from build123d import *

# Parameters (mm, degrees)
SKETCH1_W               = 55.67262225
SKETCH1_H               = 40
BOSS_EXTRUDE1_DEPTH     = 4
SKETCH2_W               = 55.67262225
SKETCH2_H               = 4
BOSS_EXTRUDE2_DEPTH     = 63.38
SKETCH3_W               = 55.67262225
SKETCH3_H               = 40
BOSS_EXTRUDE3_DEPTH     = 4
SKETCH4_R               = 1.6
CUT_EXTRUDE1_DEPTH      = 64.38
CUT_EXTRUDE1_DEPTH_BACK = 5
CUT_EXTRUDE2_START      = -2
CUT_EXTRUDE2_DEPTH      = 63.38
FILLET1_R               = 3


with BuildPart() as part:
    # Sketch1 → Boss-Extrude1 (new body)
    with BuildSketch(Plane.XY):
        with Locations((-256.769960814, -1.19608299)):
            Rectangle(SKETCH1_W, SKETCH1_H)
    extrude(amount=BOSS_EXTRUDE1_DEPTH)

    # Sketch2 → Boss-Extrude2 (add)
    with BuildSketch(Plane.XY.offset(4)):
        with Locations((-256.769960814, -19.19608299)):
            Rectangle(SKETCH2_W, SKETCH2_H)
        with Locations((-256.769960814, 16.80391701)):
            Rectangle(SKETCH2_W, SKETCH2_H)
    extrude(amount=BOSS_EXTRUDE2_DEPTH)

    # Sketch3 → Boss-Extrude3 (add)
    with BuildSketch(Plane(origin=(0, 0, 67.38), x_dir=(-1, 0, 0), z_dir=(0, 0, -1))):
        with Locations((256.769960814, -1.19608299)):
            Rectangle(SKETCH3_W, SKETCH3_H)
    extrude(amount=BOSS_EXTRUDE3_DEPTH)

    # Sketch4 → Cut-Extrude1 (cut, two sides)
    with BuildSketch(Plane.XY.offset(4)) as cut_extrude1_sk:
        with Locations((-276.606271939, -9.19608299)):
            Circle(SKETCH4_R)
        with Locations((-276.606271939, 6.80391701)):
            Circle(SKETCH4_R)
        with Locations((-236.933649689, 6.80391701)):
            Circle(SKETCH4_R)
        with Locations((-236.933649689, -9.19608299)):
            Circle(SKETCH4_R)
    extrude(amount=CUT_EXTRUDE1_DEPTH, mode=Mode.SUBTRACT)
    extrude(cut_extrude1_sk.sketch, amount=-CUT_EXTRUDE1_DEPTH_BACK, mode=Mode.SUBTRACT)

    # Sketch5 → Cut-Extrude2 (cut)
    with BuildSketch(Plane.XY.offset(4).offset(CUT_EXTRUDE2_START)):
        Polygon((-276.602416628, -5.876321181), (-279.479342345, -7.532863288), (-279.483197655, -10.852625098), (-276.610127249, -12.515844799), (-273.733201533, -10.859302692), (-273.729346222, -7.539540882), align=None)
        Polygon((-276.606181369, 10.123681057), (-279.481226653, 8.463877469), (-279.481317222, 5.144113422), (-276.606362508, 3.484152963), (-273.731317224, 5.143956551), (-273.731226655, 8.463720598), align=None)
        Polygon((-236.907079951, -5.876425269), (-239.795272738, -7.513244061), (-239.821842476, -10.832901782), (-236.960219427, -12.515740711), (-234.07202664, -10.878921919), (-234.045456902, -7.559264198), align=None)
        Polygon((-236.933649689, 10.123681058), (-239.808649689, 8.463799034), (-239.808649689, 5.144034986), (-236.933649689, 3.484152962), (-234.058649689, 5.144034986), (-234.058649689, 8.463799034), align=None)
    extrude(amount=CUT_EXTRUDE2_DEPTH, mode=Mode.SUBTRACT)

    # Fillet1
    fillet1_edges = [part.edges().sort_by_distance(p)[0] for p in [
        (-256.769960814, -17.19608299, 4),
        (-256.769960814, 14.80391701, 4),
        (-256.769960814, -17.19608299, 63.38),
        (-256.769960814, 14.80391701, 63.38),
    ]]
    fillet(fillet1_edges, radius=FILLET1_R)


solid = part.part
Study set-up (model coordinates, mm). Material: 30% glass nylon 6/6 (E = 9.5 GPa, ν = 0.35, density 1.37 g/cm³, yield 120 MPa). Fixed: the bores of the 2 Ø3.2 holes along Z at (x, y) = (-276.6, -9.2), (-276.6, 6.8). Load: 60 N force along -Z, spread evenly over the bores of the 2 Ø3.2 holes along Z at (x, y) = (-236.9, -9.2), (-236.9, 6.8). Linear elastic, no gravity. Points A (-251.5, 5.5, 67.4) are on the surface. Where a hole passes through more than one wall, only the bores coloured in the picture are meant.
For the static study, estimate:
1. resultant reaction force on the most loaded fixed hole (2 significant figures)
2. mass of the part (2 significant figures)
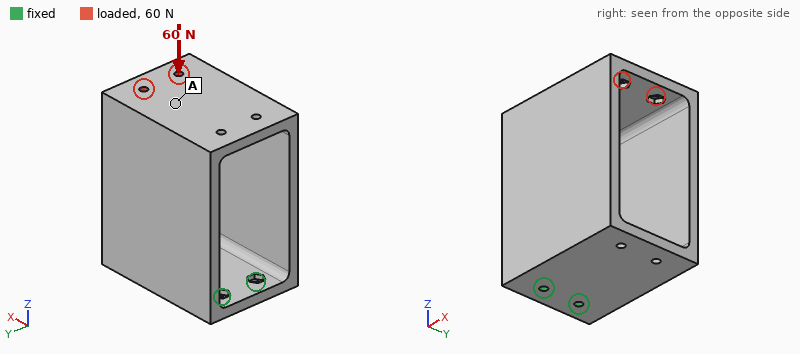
32 N
60 g
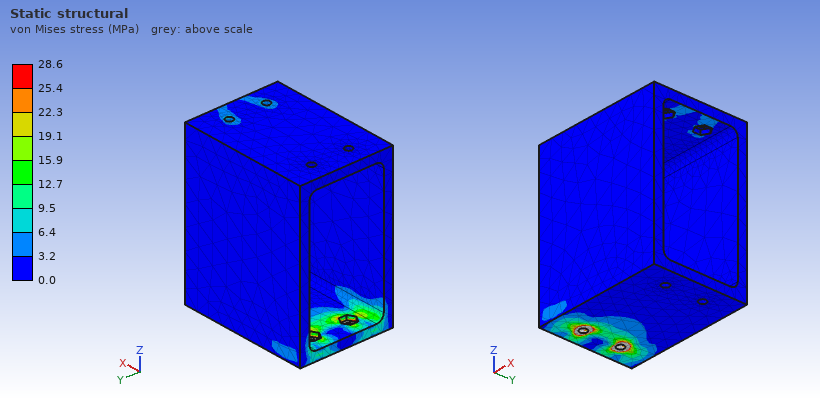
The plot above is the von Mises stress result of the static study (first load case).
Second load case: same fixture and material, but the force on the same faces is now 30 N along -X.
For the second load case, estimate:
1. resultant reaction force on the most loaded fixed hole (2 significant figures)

33 N
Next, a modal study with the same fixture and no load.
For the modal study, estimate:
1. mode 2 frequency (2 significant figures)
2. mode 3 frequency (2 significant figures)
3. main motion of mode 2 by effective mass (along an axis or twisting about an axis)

290 Hz
890 Hz
along Y
